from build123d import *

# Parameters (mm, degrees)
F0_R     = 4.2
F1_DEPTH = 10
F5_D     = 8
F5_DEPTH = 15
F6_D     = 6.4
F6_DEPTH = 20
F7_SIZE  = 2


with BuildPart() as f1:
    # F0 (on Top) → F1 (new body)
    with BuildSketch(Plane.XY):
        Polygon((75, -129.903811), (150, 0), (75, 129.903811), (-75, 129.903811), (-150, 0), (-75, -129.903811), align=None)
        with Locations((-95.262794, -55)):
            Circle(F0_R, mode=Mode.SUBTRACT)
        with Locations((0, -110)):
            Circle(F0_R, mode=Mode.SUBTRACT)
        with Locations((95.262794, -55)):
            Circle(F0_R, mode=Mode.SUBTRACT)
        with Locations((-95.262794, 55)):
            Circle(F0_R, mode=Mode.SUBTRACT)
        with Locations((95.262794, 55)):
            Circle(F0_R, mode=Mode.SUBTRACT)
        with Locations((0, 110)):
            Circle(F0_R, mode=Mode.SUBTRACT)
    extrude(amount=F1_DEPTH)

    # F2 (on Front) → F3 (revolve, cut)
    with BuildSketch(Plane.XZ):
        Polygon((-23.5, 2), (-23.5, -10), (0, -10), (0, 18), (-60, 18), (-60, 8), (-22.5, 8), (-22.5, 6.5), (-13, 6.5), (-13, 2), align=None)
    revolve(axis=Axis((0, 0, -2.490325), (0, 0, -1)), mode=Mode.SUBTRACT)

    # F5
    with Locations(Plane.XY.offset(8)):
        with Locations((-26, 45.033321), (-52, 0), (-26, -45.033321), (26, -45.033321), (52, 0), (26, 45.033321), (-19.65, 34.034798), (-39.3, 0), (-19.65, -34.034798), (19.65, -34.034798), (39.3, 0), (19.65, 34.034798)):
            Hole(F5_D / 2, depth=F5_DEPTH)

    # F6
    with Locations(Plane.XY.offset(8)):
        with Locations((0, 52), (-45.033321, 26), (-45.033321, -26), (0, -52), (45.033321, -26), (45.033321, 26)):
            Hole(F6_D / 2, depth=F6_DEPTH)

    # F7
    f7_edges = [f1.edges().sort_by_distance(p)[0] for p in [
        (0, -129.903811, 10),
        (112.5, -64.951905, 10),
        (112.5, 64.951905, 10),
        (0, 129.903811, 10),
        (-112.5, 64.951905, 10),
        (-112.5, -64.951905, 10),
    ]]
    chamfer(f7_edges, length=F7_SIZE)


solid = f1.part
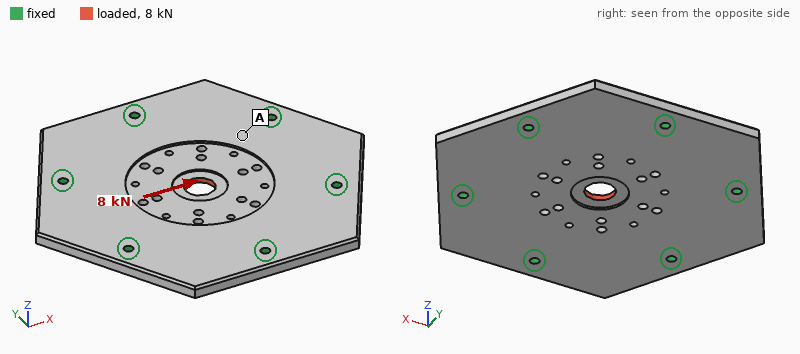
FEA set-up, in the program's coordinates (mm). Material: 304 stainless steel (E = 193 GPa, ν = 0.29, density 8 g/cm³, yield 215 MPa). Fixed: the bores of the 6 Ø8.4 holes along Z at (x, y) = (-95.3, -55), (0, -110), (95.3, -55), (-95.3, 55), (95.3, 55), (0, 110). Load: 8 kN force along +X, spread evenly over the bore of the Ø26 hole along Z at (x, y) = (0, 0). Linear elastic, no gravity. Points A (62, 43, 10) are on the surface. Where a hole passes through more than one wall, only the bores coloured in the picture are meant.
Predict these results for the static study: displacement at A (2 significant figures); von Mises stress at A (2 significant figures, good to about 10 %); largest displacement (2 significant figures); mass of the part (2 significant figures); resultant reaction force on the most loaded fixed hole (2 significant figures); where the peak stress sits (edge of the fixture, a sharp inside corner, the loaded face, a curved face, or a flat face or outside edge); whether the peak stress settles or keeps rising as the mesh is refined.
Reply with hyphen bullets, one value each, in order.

- 0.77 µm
- 3.3 MPa
- 4.2 µm
- 4.3 kg
- 1.7 kN
- a sharp inside corner
- keeps rising
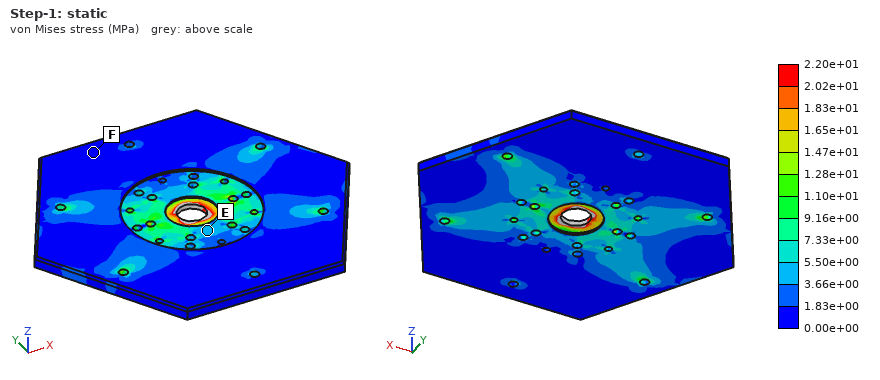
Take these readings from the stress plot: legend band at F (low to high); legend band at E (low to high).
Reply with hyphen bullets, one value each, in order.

- 0.00e+00 to 1.83e+00 MPa
- 3.66e+00 to 5.50e+00 MPa
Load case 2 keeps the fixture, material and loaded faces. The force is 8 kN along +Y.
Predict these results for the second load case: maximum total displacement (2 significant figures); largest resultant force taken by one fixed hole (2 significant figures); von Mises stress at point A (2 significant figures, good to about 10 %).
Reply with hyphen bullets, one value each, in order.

- 4.2 µm
- 2.0 kN
- 1.9 MPa
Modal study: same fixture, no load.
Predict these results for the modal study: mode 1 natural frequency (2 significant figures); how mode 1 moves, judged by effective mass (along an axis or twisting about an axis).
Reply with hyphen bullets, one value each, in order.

- 1500 Hz
- along Z
